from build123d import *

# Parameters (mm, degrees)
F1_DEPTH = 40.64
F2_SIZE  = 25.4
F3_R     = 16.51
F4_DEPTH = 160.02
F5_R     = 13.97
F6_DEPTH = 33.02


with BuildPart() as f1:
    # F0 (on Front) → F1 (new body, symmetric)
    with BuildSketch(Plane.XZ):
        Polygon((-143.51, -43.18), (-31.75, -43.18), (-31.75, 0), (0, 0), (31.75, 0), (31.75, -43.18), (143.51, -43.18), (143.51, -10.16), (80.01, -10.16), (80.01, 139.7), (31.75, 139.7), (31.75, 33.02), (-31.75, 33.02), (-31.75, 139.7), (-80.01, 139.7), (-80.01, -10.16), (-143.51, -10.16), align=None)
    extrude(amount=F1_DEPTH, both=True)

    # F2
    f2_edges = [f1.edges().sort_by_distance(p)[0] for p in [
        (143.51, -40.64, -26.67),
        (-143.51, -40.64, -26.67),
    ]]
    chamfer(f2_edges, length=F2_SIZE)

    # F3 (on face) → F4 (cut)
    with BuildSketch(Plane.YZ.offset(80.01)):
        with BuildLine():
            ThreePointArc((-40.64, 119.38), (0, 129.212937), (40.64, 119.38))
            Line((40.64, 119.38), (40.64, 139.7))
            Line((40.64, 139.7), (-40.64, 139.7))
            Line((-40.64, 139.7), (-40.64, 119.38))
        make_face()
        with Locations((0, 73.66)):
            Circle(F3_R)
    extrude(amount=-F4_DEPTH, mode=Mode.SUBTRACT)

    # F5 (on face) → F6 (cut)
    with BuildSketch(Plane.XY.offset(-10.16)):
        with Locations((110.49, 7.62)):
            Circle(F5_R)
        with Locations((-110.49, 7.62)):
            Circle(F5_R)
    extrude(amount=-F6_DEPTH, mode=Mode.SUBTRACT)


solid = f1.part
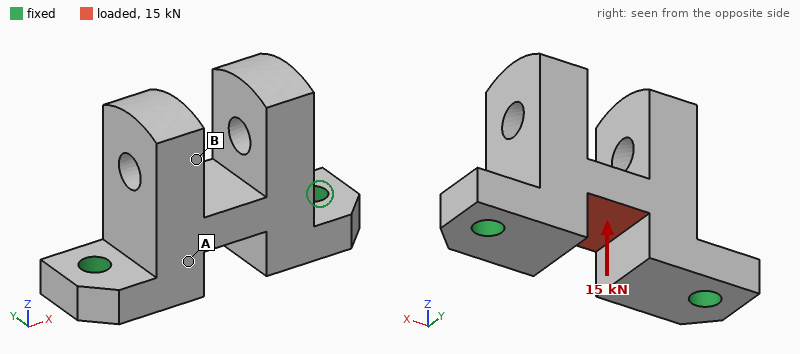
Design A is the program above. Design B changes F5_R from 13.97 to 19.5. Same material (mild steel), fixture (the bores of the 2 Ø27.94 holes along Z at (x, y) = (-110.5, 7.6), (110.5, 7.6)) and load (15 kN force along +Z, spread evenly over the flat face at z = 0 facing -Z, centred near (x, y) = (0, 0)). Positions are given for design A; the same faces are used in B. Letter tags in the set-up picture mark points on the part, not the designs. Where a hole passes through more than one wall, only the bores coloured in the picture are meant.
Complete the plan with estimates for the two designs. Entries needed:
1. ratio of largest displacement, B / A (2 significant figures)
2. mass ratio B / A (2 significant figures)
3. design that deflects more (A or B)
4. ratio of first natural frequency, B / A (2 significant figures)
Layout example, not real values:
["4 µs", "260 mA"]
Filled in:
["0.84", "0.98", "A", "1.1"]
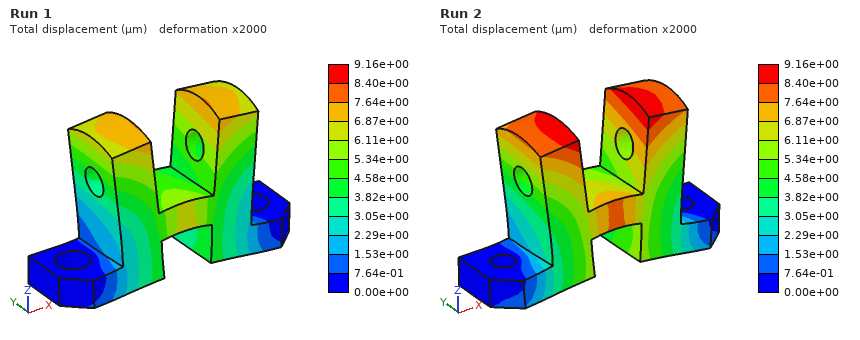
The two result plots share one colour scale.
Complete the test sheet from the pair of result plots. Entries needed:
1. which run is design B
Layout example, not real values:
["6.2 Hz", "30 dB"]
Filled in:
["Run 1"]
